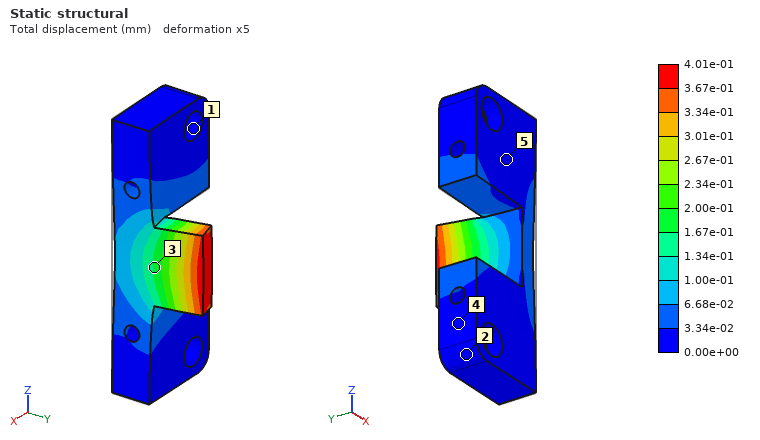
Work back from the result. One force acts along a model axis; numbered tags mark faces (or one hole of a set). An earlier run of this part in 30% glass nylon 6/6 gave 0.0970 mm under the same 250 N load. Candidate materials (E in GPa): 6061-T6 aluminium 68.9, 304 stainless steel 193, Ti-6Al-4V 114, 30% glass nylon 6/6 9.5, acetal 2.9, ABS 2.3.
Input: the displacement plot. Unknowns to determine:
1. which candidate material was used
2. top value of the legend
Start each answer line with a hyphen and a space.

- ABS
- 4.01e-01 mm
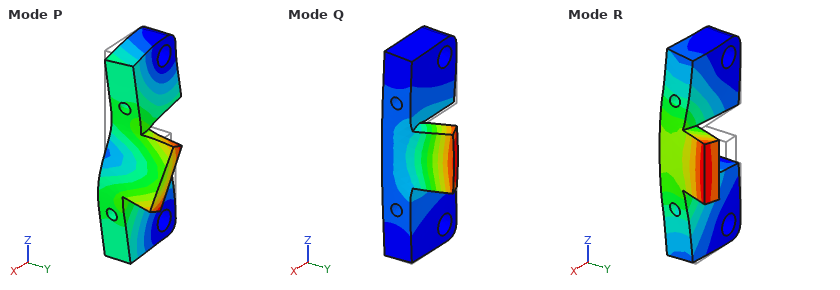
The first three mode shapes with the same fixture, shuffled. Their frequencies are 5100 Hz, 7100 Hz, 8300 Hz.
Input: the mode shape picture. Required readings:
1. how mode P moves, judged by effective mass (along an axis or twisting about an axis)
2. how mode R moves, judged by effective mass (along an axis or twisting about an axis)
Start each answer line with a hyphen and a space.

- along Z
- along Y
